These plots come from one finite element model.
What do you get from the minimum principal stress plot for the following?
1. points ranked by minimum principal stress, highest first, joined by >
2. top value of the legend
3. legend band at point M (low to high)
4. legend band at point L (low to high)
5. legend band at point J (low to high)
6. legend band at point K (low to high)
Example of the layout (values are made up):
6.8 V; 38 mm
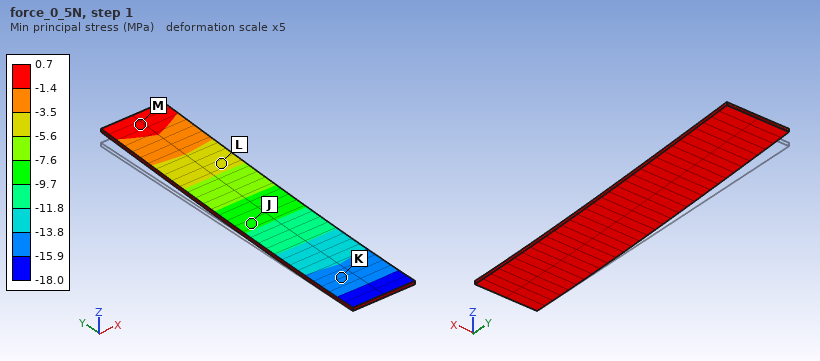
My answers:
M > L > J > K; 0.7 MPa; -1.4 to 0.7 MPa; -5.6 to -3.5 MPa; -9.7 to -7.6 MPa; -15.9 to -13.8 MPa
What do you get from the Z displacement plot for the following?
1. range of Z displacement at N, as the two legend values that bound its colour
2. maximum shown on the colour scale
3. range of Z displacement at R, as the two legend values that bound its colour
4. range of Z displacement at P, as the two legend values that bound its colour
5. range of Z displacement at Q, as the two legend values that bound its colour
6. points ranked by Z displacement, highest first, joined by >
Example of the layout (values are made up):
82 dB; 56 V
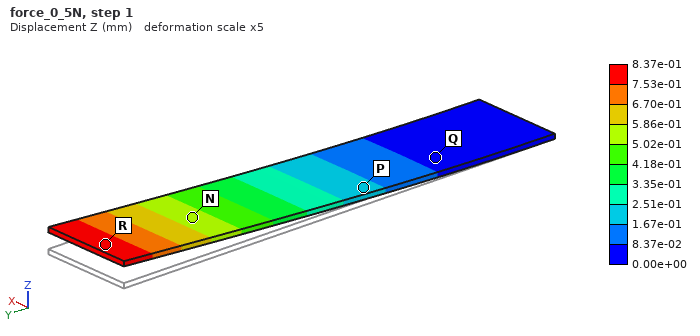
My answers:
5.02e-01 to 5.86e-01 mm; 8.37e-01 mm; 7.53e-01 to 8.37e-01 mm; 1.67e-01 to 2.51e-01 mm; 0.00e+00 to 8.37e-02 mm; R > N > P > Q
